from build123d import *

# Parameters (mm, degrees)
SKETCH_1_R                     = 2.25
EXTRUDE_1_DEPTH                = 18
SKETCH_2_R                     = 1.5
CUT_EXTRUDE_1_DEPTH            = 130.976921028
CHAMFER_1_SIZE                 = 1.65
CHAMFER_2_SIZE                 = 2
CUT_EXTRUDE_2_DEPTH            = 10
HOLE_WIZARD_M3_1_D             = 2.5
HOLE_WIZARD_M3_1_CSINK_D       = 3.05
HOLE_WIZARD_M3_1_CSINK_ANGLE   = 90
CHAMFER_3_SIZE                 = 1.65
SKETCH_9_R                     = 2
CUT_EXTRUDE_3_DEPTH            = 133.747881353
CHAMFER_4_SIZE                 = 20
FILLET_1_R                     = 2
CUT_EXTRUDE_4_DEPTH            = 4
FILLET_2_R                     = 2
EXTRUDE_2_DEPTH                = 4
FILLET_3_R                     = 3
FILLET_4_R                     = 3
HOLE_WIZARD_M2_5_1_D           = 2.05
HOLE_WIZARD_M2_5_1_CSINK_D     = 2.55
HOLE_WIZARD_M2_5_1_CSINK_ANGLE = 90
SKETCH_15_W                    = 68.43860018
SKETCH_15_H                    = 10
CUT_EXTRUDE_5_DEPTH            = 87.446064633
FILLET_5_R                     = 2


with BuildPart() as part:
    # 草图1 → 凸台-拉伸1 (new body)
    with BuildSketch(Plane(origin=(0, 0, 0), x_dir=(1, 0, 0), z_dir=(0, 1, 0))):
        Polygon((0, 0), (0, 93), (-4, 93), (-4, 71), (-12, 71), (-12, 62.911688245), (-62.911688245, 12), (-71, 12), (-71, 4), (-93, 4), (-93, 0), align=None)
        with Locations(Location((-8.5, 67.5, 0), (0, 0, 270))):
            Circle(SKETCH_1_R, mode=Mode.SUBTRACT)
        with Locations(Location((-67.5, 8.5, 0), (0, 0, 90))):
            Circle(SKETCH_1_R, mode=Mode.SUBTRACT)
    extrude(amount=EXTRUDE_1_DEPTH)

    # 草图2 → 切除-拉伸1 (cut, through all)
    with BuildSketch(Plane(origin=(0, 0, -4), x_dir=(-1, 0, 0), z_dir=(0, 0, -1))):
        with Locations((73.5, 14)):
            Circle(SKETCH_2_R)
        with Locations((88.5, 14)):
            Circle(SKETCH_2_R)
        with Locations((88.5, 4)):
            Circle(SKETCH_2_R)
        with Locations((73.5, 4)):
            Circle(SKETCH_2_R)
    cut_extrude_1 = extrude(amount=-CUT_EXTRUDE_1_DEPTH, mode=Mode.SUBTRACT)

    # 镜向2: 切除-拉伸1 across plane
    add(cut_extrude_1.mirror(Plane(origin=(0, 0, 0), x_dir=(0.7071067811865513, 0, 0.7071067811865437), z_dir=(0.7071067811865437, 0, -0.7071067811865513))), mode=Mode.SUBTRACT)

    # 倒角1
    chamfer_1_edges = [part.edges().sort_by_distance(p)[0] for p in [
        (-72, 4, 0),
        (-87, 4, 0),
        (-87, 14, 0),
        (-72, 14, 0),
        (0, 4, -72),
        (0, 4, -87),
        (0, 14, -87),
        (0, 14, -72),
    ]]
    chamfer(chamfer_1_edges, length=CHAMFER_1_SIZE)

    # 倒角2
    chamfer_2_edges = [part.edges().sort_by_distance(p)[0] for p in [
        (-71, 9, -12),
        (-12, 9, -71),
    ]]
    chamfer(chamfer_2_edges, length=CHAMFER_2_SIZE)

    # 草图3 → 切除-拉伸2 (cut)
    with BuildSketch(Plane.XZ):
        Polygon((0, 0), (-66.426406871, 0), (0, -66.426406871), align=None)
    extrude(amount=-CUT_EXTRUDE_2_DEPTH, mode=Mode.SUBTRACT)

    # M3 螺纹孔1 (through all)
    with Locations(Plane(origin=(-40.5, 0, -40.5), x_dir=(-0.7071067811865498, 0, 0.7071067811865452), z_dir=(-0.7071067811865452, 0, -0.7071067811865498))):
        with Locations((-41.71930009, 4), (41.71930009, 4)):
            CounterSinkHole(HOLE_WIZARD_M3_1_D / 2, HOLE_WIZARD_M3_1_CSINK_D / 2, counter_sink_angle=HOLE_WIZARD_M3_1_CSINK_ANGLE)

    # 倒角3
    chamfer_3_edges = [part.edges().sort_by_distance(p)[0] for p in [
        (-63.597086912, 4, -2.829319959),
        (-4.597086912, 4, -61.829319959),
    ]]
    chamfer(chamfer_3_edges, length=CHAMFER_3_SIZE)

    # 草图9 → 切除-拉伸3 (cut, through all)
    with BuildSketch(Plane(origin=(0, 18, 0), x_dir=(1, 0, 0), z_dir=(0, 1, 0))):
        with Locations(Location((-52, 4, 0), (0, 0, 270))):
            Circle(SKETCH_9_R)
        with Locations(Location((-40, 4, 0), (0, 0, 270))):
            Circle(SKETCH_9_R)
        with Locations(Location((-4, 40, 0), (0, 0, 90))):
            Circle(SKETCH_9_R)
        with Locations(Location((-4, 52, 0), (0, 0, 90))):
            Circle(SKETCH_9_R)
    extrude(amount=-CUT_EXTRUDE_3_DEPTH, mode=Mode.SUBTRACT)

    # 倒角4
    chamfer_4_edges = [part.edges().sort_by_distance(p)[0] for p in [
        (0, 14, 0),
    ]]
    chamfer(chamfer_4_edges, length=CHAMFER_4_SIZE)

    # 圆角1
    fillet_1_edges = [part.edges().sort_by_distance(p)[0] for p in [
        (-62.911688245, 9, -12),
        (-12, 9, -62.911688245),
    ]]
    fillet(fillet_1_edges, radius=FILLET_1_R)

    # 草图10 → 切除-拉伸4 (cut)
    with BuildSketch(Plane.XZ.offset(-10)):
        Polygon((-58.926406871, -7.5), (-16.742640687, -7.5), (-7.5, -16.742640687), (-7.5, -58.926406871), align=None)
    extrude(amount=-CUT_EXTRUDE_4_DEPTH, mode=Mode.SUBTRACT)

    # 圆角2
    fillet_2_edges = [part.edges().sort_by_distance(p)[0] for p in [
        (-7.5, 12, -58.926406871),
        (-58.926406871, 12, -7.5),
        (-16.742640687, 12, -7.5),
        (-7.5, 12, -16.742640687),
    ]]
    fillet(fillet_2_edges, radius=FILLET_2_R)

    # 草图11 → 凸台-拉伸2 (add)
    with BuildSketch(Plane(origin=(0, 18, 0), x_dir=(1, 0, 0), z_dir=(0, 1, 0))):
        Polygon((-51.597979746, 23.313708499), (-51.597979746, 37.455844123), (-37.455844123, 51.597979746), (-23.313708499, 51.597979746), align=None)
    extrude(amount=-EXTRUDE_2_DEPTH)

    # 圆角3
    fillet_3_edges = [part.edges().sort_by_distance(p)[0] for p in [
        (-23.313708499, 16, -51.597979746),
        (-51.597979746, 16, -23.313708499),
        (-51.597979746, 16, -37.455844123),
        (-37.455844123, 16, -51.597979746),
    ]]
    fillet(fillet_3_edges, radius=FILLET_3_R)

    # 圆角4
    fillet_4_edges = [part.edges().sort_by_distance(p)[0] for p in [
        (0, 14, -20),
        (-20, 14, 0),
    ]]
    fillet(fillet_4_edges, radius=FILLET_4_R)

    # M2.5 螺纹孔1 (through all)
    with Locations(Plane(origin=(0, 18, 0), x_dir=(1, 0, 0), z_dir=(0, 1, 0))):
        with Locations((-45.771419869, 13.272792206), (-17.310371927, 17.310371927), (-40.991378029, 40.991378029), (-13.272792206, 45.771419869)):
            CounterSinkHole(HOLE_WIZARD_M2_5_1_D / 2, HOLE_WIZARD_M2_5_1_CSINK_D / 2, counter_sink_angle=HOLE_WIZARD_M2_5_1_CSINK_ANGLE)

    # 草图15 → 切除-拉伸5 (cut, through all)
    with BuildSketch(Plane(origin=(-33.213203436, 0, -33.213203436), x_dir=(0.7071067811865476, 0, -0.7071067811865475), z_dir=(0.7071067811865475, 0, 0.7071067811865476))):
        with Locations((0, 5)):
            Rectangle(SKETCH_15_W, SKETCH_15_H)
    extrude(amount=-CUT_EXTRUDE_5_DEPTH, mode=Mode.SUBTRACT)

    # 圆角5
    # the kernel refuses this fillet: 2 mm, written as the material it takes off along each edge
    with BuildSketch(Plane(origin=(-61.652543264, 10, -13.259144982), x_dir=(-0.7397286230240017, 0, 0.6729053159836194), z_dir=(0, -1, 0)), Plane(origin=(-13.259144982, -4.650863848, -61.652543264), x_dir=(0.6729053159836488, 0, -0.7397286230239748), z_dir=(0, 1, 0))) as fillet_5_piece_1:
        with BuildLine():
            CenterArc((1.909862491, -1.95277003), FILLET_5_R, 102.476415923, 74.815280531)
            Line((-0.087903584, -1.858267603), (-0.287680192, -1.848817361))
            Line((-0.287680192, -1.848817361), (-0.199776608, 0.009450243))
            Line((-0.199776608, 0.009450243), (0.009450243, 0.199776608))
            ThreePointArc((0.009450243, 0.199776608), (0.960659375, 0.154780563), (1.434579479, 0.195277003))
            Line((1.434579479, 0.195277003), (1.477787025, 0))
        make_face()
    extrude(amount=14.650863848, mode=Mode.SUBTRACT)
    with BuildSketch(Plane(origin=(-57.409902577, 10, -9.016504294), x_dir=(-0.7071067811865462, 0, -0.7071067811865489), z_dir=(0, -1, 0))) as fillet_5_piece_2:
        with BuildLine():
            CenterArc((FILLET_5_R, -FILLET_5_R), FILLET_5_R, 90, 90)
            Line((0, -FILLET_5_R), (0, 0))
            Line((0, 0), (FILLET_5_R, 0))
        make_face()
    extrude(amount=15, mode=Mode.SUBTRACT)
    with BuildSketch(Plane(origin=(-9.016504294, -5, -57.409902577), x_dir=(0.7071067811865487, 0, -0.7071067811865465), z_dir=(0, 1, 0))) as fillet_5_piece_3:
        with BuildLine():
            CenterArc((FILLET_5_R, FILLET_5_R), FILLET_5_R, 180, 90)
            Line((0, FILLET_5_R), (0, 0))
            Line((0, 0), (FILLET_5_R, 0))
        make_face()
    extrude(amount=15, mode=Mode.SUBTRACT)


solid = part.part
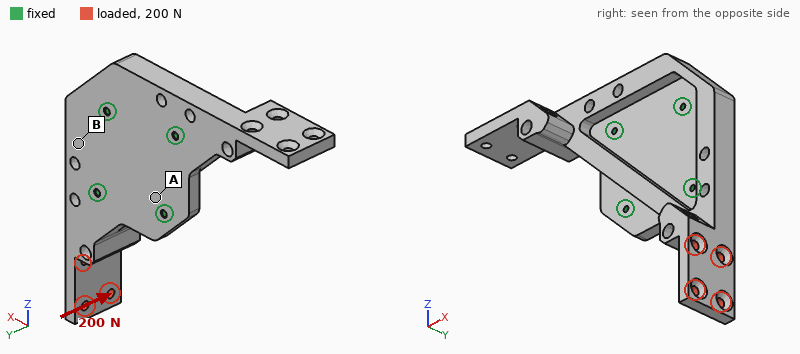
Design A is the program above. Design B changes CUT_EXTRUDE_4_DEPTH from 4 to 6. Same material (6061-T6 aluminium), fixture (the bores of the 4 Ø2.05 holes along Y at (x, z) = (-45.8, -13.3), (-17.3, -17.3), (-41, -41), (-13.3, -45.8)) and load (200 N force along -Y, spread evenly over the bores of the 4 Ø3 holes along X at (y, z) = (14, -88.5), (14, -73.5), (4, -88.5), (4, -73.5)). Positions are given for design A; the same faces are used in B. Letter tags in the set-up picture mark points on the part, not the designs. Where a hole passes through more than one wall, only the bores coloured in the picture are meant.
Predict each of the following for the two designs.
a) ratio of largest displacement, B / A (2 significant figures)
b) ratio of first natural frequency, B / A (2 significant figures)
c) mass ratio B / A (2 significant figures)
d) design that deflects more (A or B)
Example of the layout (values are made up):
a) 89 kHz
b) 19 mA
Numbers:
a) 1.3
b) 0.85
c) 0.88
d) B
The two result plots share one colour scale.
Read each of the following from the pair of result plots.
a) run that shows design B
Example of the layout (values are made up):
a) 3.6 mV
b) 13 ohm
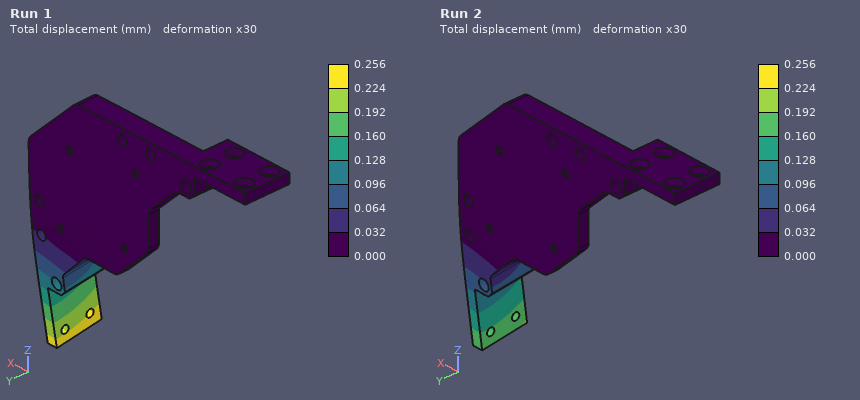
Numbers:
a) Run 1
